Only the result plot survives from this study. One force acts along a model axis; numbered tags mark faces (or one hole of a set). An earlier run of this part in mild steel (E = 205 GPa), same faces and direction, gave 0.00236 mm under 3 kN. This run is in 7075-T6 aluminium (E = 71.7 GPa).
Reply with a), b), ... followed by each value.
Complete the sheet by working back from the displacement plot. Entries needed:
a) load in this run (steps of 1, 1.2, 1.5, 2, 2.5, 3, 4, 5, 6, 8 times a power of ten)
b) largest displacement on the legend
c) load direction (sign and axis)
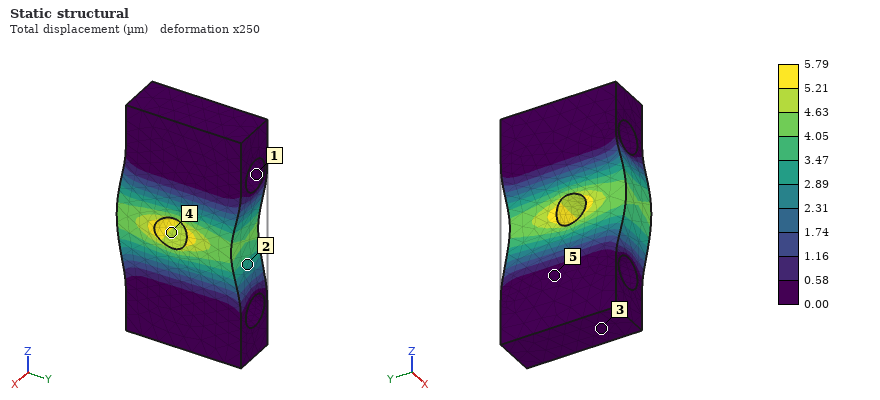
a) 2.5 kN
b) 5.79 µm
c) -Y
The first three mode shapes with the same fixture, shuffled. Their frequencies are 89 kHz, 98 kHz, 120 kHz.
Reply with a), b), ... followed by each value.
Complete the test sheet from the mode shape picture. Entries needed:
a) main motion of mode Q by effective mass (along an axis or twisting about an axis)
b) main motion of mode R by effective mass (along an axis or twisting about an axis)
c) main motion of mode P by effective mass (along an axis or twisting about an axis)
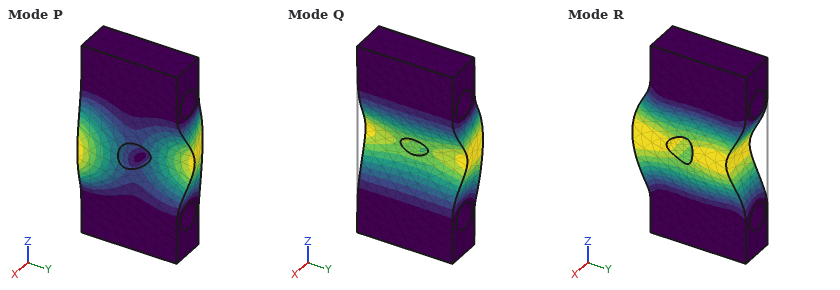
a) along X
b) along Y
c) twisting about Z
